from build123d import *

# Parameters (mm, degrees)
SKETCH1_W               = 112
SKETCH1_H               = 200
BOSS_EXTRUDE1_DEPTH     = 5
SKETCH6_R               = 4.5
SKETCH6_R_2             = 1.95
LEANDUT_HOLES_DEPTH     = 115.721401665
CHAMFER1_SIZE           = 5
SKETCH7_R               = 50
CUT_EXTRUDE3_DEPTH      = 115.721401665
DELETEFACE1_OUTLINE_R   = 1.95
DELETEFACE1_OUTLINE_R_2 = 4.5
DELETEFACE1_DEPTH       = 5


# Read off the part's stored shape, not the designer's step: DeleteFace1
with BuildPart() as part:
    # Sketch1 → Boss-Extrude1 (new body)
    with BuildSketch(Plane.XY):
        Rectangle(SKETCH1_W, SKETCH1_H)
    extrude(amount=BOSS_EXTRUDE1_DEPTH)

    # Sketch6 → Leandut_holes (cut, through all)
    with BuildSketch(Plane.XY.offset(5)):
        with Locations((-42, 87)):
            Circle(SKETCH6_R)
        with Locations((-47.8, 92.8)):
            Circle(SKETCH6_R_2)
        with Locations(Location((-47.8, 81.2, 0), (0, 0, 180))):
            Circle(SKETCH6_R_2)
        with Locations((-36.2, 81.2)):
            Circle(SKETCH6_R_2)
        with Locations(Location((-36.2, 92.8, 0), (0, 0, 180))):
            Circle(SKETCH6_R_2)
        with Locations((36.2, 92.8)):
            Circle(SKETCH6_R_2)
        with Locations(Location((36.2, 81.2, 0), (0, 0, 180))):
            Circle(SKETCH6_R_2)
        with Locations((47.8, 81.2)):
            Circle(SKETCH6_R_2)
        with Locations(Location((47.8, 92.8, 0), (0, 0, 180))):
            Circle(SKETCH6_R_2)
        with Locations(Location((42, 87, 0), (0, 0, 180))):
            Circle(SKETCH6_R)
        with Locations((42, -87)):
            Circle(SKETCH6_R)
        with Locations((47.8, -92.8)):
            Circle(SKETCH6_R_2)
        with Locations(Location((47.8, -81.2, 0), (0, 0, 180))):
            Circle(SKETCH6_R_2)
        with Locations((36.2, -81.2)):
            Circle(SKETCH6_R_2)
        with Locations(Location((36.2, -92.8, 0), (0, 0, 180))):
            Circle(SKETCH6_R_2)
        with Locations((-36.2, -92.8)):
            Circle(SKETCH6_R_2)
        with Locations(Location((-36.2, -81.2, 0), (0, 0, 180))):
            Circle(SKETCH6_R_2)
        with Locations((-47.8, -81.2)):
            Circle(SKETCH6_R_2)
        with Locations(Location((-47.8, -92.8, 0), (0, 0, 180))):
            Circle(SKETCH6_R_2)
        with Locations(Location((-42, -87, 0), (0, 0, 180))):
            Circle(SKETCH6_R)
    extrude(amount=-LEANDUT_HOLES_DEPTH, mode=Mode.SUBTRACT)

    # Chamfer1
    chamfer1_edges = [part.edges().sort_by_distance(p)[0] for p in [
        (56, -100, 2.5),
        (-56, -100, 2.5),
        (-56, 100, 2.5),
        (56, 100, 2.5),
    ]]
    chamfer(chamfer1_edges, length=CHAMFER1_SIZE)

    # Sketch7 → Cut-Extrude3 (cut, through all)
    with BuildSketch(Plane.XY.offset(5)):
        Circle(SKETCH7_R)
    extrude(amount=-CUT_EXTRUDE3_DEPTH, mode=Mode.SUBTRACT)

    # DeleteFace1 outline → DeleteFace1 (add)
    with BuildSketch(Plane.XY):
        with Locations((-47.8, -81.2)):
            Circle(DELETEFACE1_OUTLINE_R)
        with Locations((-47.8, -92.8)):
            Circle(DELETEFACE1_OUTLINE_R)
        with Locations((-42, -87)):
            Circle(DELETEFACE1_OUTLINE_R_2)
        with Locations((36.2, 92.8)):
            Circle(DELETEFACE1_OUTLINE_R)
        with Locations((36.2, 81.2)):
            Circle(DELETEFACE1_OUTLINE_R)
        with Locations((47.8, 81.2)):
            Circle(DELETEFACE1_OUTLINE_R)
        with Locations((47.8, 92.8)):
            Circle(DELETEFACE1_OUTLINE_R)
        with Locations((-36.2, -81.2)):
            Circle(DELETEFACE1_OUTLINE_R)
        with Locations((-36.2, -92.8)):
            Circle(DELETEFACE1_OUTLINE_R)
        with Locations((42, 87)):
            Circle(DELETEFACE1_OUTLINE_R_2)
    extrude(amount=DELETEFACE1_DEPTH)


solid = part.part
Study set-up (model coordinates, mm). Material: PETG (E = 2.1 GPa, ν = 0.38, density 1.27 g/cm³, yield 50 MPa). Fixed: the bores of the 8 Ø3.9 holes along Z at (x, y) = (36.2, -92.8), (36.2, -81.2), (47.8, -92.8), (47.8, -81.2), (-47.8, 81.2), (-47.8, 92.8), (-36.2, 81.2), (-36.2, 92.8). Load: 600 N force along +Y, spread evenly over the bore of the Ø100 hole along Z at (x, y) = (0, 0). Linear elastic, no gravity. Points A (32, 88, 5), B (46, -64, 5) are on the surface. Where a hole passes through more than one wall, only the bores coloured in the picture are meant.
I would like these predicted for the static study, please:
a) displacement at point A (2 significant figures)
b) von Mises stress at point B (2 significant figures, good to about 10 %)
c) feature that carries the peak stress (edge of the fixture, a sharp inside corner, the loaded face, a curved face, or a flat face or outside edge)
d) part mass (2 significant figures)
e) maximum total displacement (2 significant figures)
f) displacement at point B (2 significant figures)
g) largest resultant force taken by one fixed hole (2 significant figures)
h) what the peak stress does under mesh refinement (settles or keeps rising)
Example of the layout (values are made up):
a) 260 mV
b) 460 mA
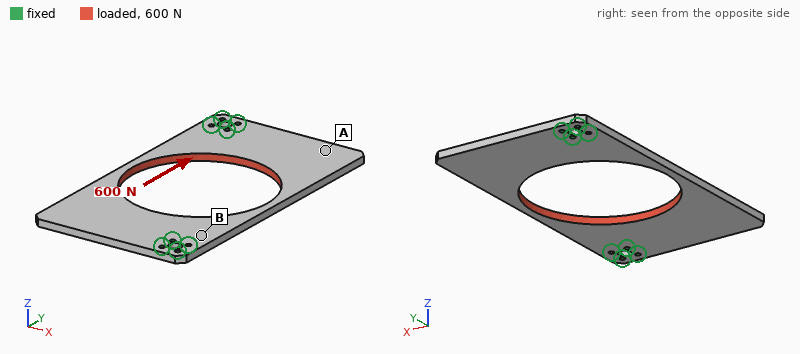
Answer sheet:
a) 0.11 mm
b) 1.9 MPa
c) edge of the fixture
d) 91 g
e) 0.14 mm
f) 0.022 mm
g) 200 N
h) keeps rising
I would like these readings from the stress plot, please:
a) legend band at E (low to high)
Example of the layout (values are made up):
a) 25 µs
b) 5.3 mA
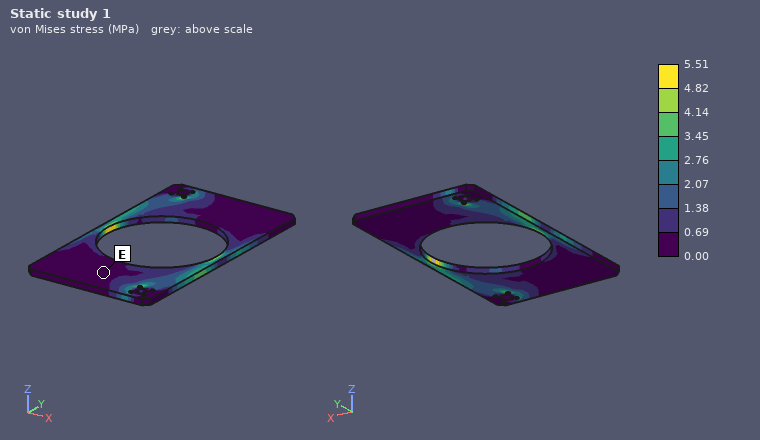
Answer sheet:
a) 0.00 to 0.69 MPa
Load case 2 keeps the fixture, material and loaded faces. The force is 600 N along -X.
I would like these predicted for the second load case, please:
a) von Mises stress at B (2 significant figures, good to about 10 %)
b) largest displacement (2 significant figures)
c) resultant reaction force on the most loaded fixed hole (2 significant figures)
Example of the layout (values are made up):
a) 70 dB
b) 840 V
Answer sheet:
a) 1.00 MPa
b) 0.23 mm
c) 220 N
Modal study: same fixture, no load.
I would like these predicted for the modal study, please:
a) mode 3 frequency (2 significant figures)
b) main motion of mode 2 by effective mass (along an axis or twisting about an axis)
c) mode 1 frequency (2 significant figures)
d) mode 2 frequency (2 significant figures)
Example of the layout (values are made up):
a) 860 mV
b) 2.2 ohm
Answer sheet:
a) 280 Hz
b) along Z
c) 120 Hz
d) 130 Hz
